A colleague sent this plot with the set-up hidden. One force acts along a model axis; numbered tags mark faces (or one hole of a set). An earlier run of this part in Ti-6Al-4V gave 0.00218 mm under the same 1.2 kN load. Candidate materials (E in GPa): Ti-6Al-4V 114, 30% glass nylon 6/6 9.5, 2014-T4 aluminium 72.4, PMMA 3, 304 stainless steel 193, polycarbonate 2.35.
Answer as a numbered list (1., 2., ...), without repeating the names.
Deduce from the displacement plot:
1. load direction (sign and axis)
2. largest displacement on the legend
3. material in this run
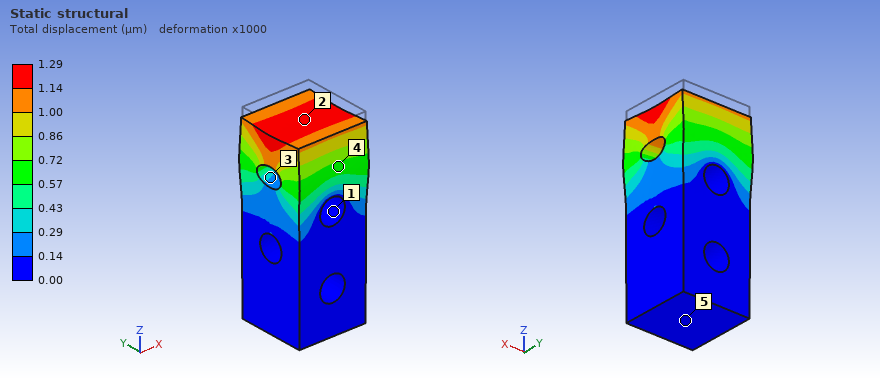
1. -Z
2. 1.29 µm
3. 304 stainless steel
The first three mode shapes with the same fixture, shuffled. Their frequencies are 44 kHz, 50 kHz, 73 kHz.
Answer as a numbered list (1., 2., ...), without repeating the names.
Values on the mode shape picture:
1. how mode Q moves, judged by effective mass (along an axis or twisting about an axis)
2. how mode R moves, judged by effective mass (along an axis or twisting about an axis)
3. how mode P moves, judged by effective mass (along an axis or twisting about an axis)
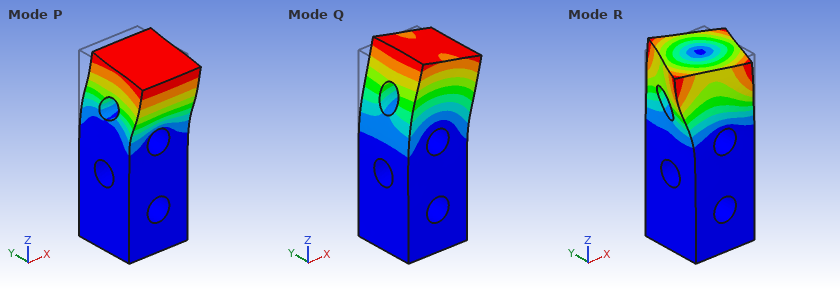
1. along X
2. twisting about Z
3. along Y
